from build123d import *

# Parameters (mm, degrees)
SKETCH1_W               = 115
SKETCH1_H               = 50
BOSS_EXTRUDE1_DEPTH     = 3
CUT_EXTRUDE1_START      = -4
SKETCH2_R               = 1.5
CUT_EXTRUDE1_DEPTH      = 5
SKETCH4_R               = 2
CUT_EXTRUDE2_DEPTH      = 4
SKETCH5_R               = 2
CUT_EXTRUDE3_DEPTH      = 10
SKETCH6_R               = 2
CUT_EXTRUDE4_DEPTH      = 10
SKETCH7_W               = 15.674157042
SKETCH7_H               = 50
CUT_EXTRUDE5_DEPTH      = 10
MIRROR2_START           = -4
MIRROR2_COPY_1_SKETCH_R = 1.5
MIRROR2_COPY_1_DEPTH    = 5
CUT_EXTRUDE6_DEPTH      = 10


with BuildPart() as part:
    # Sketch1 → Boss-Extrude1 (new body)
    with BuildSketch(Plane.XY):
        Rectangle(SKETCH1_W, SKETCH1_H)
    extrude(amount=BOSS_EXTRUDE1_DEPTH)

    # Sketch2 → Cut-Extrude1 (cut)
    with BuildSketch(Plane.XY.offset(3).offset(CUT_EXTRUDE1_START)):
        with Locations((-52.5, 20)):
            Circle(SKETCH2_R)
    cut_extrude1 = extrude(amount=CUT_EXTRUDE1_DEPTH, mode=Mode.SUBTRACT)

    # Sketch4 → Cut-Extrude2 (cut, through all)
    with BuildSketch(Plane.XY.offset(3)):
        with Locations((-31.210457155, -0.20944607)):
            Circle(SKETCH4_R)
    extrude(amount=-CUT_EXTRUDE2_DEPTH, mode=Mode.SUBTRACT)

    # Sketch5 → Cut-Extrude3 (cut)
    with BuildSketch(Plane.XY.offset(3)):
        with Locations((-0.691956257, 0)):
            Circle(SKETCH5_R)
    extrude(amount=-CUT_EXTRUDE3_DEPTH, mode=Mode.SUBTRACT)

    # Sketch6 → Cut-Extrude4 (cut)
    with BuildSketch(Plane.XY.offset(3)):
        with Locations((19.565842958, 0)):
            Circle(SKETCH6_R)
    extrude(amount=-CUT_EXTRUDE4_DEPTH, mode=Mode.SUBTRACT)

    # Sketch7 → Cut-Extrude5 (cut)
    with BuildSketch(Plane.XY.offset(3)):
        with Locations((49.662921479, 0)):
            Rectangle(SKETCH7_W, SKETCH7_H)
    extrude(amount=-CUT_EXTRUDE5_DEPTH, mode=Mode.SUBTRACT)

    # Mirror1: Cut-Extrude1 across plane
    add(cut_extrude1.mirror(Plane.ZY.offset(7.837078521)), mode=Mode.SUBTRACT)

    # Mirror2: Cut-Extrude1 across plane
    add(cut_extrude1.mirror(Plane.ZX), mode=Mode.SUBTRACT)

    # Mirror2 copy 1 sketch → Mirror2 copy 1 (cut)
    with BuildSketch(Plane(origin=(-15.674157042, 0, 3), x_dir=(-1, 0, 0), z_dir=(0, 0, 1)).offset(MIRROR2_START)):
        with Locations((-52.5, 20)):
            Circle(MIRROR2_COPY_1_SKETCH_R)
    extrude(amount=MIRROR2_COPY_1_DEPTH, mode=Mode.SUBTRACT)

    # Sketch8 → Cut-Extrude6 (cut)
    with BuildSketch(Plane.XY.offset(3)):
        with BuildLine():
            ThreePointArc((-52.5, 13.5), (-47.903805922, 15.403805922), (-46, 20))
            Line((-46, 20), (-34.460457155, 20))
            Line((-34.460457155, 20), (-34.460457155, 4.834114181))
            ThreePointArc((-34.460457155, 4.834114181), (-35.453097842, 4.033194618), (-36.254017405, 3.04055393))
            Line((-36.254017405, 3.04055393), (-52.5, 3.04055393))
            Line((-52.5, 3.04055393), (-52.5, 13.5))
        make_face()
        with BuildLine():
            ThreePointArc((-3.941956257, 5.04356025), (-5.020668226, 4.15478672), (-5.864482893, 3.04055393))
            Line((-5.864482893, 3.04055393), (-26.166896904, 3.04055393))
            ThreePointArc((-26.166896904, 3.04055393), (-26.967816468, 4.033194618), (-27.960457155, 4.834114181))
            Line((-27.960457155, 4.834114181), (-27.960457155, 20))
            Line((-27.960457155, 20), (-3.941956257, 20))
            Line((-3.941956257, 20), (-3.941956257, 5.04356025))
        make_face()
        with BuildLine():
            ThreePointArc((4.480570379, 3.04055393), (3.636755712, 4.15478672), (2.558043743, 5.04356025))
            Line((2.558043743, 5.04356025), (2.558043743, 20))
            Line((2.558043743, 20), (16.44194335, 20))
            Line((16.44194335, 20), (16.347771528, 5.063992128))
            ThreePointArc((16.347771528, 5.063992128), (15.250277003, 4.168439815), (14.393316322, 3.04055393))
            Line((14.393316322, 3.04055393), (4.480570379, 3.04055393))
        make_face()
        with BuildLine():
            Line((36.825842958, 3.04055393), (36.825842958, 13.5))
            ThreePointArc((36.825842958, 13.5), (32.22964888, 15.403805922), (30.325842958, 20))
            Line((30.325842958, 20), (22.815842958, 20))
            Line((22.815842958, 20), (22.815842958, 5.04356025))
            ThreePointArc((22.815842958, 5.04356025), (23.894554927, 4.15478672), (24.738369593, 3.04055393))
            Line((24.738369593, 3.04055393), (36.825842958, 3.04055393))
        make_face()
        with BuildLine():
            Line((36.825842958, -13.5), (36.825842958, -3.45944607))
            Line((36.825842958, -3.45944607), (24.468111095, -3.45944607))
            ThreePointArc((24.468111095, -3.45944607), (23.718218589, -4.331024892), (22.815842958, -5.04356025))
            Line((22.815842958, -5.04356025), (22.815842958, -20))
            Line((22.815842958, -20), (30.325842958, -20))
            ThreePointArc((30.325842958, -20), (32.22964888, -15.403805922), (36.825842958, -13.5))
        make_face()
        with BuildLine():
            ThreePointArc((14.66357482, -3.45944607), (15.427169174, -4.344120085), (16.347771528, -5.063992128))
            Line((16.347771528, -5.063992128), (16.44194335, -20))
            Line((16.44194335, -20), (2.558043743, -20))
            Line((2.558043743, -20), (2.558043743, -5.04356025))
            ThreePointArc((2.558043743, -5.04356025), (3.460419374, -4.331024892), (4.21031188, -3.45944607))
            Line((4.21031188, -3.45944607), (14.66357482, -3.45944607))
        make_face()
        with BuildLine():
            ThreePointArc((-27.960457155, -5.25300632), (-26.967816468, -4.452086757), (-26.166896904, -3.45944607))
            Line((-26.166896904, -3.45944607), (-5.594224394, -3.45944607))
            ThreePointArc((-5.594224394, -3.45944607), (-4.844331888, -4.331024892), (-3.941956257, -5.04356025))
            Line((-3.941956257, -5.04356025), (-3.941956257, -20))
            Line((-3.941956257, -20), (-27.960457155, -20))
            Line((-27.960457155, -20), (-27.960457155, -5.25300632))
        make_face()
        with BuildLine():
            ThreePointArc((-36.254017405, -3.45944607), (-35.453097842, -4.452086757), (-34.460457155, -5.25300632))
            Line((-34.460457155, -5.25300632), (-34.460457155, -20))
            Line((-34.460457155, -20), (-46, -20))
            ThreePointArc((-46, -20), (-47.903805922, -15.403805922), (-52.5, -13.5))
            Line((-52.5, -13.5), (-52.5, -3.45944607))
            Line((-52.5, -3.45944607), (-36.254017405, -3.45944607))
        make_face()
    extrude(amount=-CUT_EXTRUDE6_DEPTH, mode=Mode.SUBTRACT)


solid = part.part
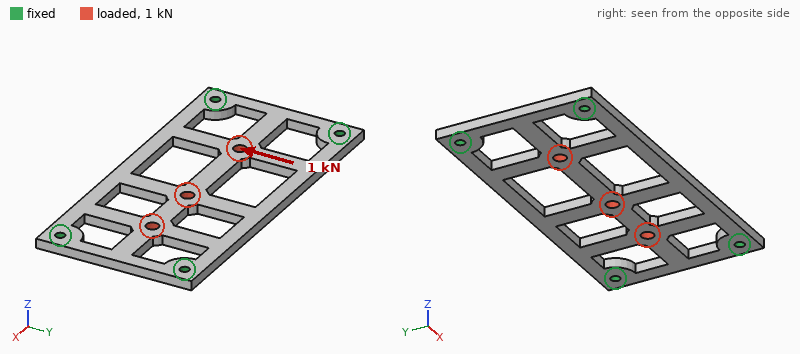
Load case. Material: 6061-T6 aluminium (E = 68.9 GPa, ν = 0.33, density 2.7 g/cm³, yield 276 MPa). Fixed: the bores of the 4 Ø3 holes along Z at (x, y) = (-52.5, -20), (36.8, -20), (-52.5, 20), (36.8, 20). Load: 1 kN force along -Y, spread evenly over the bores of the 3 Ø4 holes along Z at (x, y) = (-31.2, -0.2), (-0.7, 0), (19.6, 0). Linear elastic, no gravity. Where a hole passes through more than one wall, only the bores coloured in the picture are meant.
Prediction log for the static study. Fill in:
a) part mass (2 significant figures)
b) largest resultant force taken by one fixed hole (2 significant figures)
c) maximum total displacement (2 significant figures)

22 g
340 N
62 µm
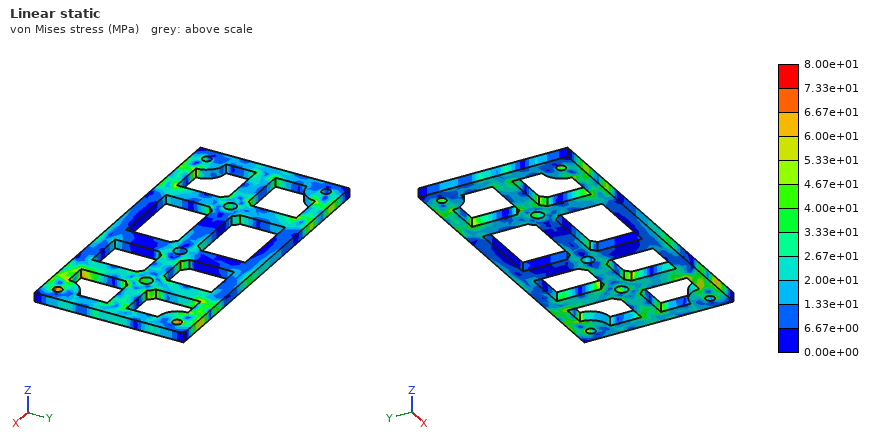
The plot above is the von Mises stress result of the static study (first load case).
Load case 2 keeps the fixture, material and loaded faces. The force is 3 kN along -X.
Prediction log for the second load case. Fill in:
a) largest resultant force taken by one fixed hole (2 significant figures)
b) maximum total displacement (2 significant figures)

810 N
72 µm
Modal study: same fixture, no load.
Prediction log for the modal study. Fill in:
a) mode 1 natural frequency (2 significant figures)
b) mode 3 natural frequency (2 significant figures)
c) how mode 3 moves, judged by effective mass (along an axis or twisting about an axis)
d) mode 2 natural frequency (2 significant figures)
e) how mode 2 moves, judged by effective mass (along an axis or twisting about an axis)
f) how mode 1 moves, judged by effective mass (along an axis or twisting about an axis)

1600 Hz
3900 Hz
twisting about Y
2600 Hz
twisting about X
along Z
